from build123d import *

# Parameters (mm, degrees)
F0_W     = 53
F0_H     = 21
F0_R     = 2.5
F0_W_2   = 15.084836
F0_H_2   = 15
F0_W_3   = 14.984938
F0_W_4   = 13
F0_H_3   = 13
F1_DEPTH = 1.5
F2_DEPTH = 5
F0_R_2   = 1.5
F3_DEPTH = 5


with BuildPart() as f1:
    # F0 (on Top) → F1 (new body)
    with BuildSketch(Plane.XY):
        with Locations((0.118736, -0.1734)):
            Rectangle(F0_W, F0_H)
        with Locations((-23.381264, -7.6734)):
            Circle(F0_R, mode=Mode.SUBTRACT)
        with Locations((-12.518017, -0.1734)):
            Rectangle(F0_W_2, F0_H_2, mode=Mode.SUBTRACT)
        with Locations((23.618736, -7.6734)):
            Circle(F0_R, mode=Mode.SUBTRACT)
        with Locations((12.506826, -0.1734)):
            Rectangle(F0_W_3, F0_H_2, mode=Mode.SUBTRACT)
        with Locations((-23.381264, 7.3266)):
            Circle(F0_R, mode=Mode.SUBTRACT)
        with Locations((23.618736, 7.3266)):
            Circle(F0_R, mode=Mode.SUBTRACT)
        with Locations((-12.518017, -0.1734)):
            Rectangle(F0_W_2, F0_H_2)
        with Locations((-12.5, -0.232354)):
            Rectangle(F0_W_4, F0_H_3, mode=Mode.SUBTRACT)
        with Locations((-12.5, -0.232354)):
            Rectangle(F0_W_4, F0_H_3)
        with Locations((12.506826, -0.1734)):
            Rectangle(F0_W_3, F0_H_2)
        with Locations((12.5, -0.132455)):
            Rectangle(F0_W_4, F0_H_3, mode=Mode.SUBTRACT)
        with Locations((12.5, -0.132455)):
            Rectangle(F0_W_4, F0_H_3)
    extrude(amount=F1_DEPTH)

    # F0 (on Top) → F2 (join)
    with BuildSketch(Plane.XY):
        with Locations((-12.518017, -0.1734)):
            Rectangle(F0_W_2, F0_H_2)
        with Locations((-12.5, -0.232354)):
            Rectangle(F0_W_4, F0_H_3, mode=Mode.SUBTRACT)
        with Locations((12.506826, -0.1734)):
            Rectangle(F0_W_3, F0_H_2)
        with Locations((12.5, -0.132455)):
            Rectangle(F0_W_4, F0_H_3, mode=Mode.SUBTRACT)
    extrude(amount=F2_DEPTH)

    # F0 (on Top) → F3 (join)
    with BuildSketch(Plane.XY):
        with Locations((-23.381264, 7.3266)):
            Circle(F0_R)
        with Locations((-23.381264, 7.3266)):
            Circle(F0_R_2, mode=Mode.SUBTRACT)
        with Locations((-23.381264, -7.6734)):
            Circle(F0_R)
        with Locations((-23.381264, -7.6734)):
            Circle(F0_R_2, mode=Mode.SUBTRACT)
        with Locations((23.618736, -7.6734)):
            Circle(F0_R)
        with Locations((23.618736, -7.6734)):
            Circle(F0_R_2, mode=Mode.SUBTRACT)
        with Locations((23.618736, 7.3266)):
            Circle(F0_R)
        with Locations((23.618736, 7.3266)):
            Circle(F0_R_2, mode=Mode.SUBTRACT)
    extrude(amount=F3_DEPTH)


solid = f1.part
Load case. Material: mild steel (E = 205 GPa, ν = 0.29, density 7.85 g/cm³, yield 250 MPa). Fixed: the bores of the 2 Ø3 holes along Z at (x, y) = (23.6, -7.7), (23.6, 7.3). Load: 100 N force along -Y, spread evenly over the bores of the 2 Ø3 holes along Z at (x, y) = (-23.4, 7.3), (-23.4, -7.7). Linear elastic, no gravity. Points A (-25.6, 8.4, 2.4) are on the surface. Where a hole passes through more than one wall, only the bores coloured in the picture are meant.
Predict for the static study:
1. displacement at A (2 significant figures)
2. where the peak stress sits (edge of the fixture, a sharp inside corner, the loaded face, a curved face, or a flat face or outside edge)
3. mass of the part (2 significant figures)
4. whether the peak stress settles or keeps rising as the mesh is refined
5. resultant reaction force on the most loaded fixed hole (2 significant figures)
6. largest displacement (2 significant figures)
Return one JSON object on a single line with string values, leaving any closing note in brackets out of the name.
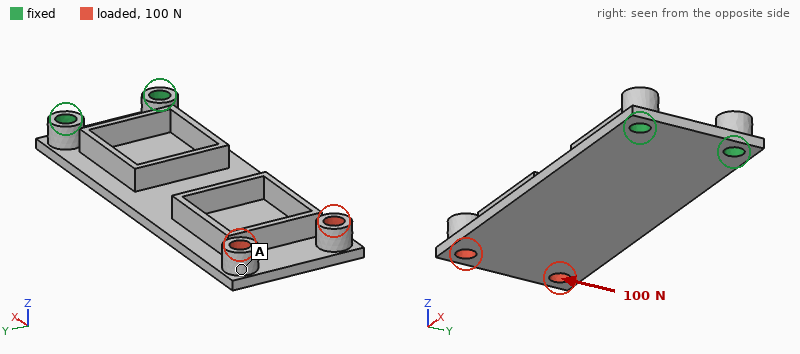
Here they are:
{"displacement at A": "34 µm", "where the peak stress sits": "edge of the fixture", "mass of the part": "17 g", "whether the peak stress settles or keeps rising as the mesh is refined": "keeps rising", "resultant reaction force on the most loaded fixed hole": "300 N", "largest displacement": "41 µm"}
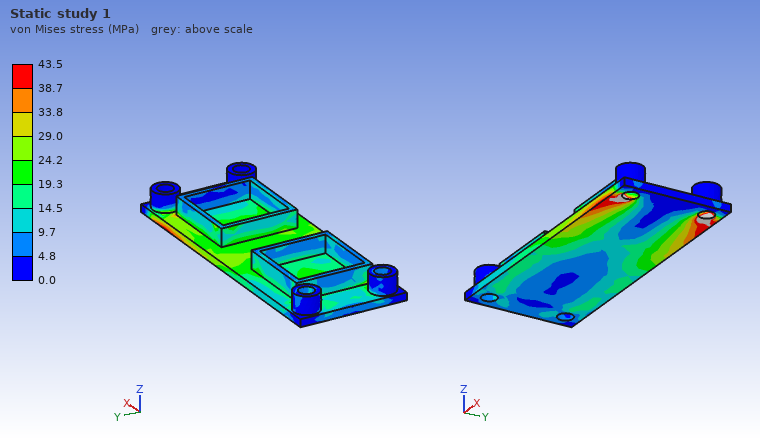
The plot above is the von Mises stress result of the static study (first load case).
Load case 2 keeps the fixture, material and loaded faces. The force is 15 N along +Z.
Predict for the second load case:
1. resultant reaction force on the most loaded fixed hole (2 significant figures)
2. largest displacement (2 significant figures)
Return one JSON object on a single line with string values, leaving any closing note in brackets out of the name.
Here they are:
{"resultant reaction force on the most loaded fixed hole": "18 N", "largest displacement": "0.23 mm"}
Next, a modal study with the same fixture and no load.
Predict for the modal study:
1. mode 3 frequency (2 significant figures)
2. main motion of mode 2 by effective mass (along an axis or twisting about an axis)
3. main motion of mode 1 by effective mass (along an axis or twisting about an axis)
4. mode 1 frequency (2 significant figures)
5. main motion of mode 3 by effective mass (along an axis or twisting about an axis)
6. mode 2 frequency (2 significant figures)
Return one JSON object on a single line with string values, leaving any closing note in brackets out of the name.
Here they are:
{"mode 3 frequency": "3400 Hz", "main motion of mode 2 by effective mass": "twisting about X", "main motion of mode 1 by effective mass": "along Z", "mode 1 frequency": "610 Hz", "main motion of mode 3 by effective mass": "along Z", "mode 2 frequency": "2500 Hz"}
